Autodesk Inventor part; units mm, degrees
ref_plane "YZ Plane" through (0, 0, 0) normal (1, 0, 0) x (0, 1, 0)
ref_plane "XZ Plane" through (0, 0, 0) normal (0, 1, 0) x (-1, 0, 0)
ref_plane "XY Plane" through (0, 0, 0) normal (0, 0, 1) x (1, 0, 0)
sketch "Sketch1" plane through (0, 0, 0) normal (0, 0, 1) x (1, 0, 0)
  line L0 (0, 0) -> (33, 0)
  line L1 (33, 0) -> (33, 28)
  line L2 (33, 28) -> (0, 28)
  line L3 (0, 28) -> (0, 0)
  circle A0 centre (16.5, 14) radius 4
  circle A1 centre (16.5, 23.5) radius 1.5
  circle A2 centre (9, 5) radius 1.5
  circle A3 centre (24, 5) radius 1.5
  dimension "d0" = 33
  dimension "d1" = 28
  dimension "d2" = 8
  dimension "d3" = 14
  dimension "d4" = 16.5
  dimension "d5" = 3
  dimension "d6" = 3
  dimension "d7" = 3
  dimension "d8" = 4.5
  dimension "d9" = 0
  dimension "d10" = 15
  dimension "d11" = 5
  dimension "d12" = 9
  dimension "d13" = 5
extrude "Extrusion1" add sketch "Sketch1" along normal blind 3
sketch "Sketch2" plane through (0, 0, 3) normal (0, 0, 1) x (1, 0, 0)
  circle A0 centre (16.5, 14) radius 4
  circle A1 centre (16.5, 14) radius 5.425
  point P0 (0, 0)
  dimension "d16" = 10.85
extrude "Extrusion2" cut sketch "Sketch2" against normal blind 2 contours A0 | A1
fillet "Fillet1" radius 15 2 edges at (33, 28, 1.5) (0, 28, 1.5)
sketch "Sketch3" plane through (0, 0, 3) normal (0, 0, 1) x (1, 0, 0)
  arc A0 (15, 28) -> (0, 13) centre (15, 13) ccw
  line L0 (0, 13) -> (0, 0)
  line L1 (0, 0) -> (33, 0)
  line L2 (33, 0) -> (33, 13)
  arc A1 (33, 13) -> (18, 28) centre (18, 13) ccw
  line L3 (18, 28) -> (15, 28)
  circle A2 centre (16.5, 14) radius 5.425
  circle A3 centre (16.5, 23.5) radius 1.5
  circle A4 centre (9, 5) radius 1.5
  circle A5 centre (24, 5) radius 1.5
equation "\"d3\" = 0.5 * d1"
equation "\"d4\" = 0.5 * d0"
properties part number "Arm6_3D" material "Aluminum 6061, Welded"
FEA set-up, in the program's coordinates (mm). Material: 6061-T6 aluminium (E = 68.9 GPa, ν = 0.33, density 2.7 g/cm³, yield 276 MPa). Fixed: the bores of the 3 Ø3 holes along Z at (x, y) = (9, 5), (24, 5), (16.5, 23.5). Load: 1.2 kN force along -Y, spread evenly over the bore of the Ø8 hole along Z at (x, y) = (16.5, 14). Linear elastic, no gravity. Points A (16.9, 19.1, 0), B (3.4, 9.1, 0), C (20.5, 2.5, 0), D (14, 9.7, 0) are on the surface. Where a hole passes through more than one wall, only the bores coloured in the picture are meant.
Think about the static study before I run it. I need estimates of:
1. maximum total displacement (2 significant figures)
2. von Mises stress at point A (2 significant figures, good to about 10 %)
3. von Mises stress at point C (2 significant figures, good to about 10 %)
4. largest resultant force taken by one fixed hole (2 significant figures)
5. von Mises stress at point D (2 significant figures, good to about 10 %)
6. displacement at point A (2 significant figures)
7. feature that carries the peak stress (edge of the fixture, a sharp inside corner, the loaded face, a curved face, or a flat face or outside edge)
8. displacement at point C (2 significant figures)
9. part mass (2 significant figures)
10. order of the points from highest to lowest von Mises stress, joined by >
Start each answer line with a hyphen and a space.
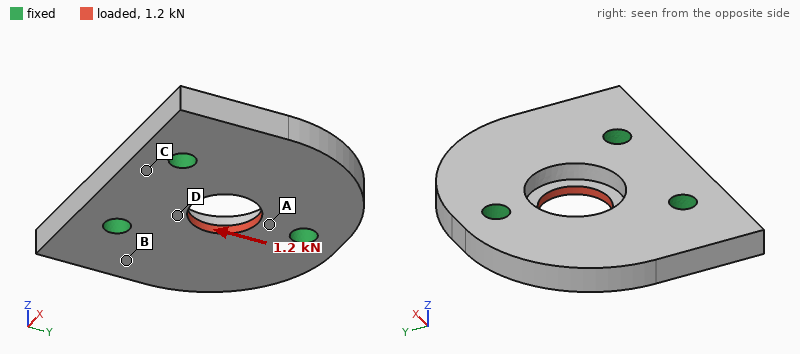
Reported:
- 5.8 µm
- 57 MPa
- 13 MPa
- 430 N
- 43 MPa
- 2.8 µm
- the loaded face
- 1.1 µm
- 5.9 g
- A > D > C > B
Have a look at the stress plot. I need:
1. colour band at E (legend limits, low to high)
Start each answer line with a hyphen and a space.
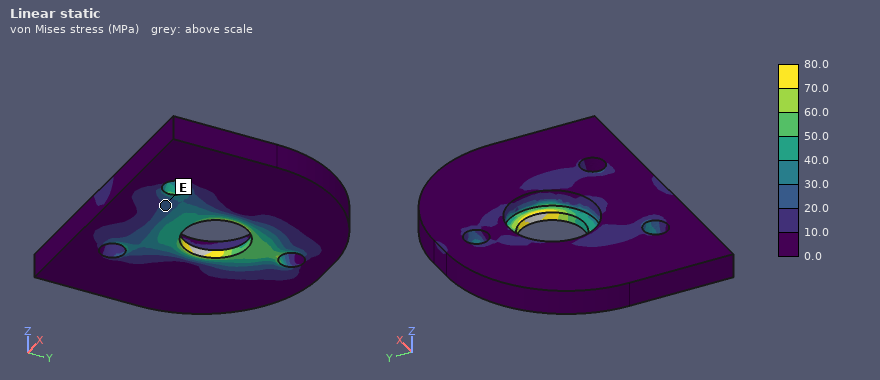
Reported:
- 20.0 to 30.0 MPa
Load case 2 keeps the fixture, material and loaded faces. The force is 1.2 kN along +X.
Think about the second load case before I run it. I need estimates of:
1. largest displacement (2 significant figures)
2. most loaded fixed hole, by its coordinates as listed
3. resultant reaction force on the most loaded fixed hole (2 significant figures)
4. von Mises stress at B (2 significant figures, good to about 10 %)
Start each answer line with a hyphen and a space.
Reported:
- 6.5 µm
- (16.5, 23.5)
- 560 N
- 10 MPa
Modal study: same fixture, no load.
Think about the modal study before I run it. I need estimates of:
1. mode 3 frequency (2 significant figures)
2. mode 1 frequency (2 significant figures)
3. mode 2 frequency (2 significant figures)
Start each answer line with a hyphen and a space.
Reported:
- 33 kHz
- 16 kHz
- 17 kHz
